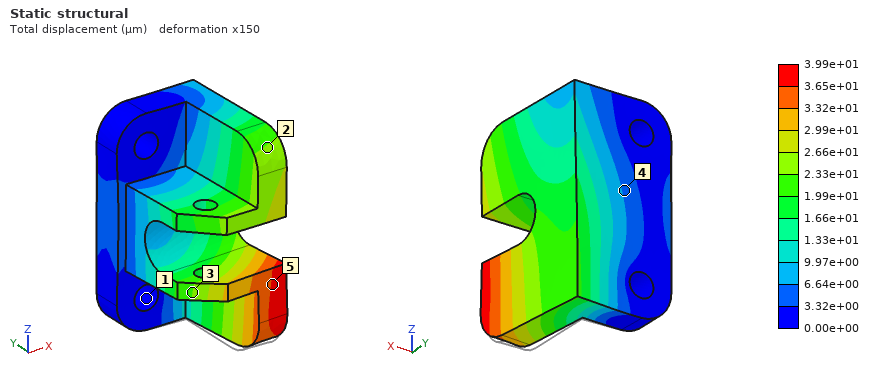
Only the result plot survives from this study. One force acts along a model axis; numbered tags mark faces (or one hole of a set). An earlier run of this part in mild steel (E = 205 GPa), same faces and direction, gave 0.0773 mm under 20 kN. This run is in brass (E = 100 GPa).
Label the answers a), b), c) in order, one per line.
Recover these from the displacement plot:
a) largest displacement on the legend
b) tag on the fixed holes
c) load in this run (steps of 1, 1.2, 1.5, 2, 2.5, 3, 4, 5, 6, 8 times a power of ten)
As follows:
a) 3.99e+01 µm
b) 1
c) 5 kN
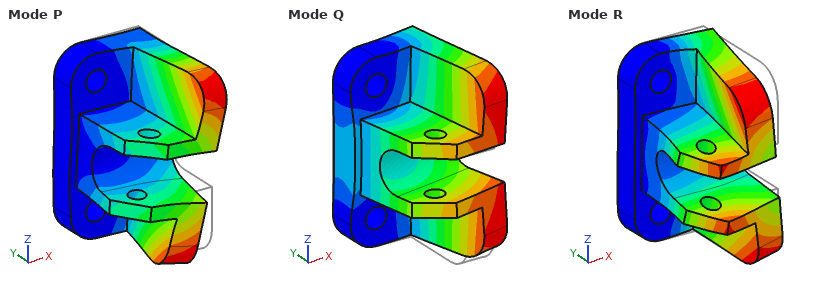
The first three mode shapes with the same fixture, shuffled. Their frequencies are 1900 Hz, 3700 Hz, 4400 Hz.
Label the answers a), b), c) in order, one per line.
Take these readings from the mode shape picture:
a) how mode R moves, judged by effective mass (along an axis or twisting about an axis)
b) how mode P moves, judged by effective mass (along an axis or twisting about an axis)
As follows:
a) along Z
b) along Z
